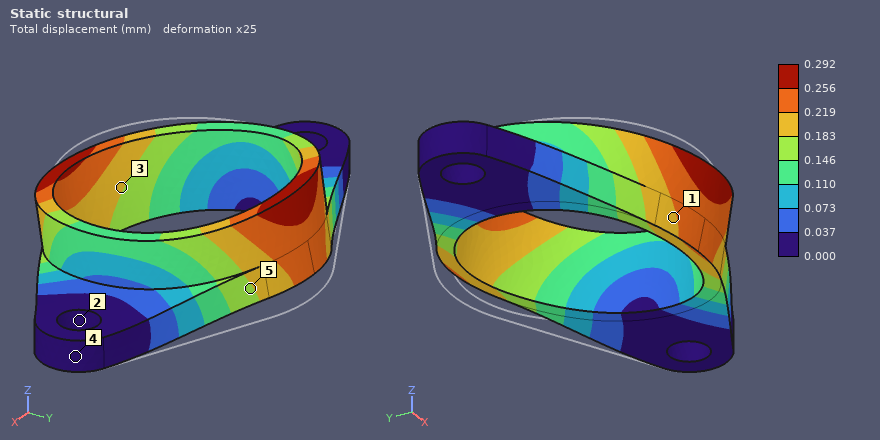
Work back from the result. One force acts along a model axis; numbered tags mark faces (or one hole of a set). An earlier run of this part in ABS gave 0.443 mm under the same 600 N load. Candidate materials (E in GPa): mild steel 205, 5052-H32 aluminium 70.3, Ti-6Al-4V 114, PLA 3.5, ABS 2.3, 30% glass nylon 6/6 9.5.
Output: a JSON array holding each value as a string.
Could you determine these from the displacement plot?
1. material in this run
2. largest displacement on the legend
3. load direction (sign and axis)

["PLA", "0.292 mm", "-Y"]
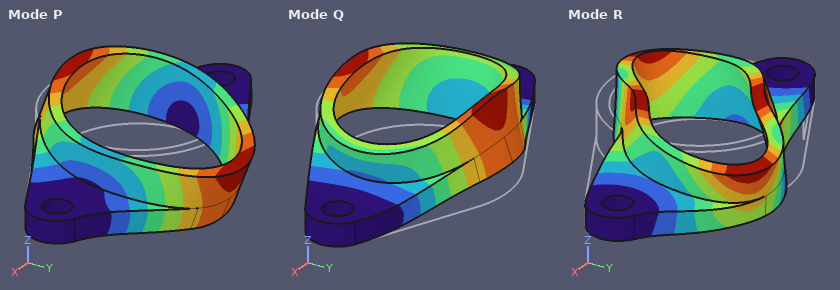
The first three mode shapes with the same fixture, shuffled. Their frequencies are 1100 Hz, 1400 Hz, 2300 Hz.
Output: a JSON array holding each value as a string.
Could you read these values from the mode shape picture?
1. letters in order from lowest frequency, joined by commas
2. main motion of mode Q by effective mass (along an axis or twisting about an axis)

["P, Q, R", "along Z"]
